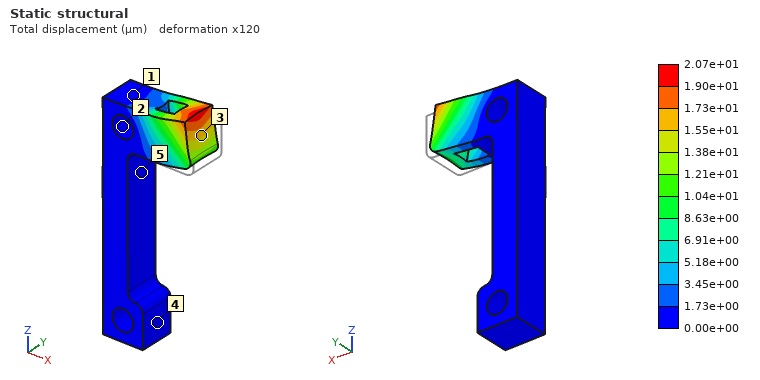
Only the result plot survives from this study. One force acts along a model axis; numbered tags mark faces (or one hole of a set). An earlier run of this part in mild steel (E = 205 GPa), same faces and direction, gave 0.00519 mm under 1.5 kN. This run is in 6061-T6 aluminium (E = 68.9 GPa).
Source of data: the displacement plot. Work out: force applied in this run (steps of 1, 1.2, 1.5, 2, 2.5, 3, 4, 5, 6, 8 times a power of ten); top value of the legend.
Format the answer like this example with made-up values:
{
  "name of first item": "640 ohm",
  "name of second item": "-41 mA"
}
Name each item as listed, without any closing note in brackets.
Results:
{
  "force applied in this run": "2 kN",
  "top value of the legend": "2.07e+01 µm"
}
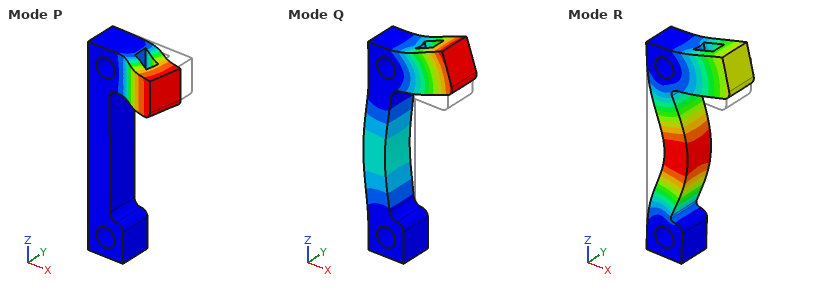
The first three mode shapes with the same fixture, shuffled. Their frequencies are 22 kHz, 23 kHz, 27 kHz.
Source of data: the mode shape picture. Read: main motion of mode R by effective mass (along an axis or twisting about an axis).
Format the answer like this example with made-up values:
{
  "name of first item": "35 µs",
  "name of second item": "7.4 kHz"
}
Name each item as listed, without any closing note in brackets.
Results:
{
  "main motion of mode R by effective mass": "along X"
}
